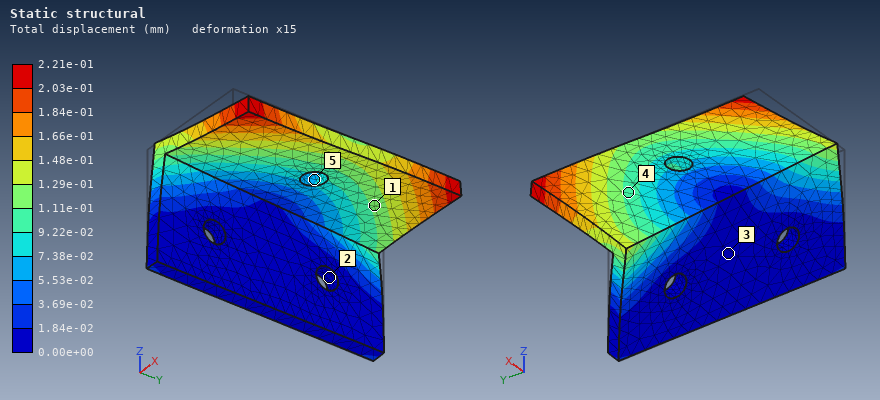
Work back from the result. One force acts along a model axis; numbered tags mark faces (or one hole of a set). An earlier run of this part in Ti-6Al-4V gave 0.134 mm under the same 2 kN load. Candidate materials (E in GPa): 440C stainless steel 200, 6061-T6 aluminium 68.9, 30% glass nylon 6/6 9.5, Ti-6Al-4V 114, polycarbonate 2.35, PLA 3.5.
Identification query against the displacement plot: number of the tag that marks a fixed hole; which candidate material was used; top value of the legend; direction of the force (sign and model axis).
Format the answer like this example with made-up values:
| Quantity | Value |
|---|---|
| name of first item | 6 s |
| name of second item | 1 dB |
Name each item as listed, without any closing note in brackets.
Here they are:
| Quantity | Value |
|---|---|
| number of the tag that marks a fixed hole | 2 |
| which candidate material was used | 6061-T6 aluminium |
| top value of the legend | 2.21e-01 mm |
| direction of the force | +Y |
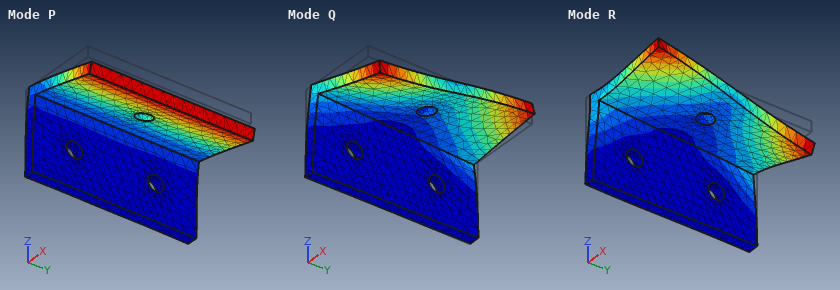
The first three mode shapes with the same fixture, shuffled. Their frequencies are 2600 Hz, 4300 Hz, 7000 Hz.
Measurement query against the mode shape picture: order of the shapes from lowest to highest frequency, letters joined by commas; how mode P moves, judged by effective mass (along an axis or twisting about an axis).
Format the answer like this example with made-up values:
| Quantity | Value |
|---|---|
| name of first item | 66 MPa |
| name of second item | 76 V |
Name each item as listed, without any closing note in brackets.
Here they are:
| Quantity | Value |
|---|---|
| order of the shapes from lowest to highest frequency, letters joined by commas | P, Q, R |
| how mode P moves, judged by effective mass | along Z |
